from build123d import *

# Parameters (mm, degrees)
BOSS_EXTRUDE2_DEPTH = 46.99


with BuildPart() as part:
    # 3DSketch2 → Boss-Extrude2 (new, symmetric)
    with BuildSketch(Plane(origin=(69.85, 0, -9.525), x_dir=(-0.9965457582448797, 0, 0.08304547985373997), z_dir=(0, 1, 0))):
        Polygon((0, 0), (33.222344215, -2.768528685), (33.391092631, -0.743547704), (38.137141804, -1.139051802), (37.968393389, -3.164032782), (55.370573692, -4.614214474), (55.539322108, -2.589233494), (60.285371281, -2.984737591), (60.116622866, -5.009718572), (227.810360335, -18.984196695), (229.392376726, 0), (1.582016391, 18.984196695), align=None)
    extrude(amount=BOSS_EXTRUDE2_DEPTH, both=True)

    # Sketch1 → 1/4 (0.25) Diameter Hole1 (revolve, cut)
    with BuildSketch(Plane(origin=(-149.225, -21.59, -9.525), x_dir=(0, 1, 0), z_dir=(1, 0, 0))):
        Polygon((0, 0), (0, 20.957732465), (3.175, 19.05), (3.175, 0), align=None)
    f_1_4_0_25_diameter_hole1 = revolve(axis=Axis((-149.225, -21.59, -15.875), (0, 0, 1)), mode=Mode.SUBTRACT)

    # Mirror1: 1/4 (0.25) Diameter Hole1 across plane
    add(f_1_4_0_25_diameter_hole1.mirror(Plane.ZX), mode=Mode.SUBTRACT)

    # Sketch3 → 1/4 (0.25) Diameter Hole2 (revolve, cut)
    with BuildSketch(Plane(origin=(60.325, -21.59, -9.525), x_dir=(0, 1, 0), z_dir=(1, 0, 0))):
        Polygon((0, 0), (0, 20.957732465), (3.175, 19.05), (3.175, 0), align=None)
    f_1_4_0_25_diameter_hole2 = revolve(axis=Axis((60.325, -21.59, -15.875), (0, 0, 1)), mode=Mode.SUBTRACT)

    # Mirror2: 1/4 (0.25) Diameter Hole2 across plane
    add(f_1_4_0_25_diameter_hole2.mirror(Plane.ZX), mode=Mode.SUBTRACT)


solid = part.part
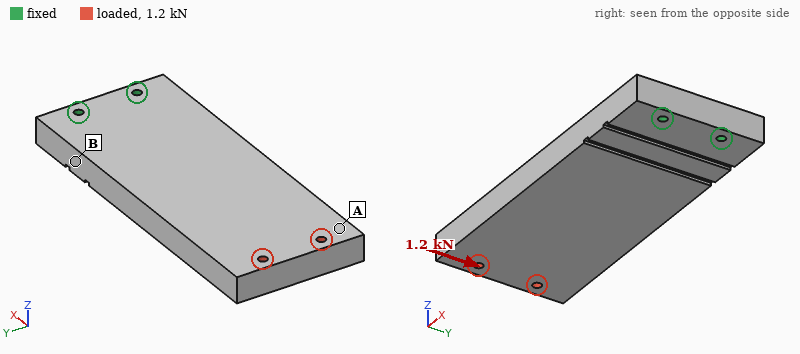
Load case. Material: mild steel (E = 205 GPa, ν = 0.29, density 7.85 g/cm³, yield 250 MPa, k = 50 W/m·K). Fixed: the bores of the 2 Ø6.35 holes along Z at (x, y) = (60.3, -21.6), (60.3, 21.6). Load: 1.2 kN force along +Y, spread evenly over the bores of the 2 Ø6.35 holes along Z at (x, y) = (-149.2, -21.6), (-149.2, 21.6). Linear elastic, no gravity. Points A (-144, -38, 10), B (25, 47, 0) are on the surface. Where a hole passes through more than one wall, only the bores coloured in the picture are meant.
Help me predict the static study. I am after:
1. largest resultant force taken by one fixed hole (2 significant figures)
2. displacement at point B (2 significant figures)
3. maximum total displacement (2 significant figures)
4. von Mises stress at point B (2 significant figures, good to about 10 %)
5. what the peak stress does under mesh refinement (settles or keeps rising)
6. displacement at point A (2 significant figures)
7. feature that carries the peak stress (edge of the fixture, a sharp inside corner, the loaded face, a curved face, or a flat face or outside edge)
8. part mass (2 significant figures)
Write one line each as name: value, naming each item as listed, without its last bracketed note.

largest resultant force taken by one fixed hole: 5.3 kN
displacement at point B: 4.5 µm
maximum total displacement: 27 µm
von Mises stress at point B: 7.1 MPa
what the peak stress does under mesh refinement: keeps rising
displacement at point A: 25 µm
feature that carries the peak stress: edge of the fixture
part mass: 3.2 kg
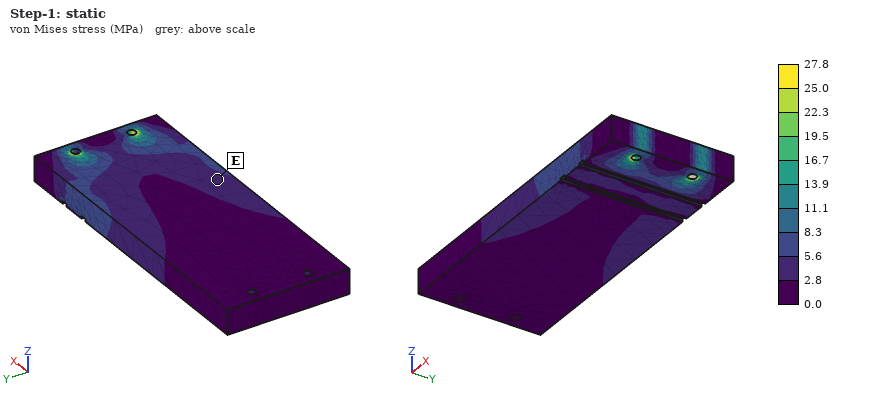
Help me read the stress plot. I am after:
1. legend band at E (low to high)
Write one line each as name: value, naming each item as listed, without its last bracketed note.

legend band at E: 2.8 to 5.6 MPa
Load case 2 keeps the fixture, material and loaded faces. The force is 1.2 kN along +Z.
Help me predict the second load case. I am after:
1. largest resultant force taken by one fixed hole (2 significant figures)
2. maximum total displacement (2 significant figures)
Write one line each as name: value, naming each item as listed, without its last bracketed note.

largest resultant force taken by one fixed hole: 600 N
maximum total displacement: 0.42 mm
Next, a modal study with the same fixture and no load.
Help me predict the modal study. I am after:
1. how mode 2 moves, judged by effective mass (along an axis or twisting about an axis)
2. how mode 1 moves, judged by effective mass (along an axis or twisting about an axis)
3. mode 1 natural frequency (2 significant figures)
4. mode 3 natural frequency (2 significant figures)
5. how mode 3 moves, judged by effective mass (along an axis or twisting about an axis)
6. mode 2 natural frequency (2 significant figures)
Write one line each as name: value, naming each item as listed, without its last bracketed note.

how mode 2 moves, judged by effective mass: along Y
how mode 1 moves, judged by effective mass: along Z
mode 1 natural frequency: 300 Hz
mode 3 natural frequency: 1400 Hz
how mode 3 moves, judged by effective mass: twisting about X
mode 2 natural frequency: 1100 Hz
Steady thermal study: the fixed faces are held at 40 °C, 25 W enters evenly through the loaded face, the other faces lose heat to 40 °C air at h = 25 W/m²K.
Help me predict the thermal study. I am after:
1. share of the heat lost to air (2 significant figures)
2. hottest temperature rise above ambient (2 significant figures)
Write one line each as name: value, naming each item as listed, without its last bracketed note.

share of the heat lost to air: 70 %
hottest temperature rise above ambient: 32 K
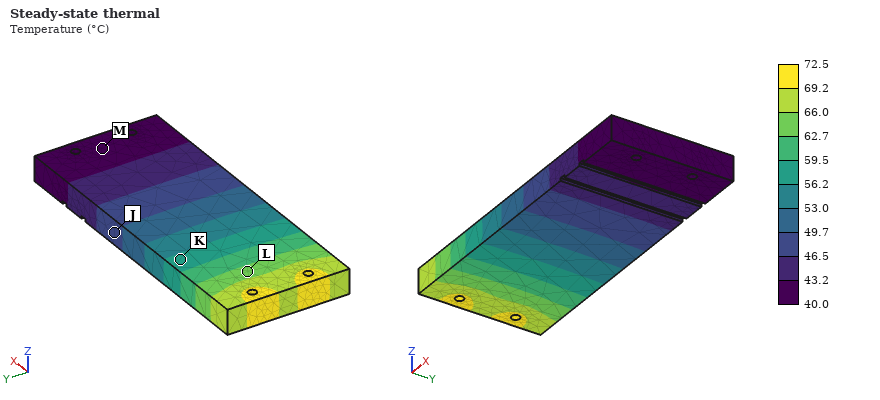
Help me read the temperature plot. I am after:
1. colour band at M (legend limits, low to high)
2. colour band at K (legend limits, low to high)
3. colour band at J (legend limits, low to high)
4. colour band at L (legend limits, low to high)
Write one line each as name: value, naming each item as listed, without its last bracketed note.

colour band at M: 40.0 to 43.2 °C
colour band at K: 56.2 to 59.5 °C
colour band at J: 46.5 to 49.7 °C
colour band at L: 62.7 to 66.0 °C
